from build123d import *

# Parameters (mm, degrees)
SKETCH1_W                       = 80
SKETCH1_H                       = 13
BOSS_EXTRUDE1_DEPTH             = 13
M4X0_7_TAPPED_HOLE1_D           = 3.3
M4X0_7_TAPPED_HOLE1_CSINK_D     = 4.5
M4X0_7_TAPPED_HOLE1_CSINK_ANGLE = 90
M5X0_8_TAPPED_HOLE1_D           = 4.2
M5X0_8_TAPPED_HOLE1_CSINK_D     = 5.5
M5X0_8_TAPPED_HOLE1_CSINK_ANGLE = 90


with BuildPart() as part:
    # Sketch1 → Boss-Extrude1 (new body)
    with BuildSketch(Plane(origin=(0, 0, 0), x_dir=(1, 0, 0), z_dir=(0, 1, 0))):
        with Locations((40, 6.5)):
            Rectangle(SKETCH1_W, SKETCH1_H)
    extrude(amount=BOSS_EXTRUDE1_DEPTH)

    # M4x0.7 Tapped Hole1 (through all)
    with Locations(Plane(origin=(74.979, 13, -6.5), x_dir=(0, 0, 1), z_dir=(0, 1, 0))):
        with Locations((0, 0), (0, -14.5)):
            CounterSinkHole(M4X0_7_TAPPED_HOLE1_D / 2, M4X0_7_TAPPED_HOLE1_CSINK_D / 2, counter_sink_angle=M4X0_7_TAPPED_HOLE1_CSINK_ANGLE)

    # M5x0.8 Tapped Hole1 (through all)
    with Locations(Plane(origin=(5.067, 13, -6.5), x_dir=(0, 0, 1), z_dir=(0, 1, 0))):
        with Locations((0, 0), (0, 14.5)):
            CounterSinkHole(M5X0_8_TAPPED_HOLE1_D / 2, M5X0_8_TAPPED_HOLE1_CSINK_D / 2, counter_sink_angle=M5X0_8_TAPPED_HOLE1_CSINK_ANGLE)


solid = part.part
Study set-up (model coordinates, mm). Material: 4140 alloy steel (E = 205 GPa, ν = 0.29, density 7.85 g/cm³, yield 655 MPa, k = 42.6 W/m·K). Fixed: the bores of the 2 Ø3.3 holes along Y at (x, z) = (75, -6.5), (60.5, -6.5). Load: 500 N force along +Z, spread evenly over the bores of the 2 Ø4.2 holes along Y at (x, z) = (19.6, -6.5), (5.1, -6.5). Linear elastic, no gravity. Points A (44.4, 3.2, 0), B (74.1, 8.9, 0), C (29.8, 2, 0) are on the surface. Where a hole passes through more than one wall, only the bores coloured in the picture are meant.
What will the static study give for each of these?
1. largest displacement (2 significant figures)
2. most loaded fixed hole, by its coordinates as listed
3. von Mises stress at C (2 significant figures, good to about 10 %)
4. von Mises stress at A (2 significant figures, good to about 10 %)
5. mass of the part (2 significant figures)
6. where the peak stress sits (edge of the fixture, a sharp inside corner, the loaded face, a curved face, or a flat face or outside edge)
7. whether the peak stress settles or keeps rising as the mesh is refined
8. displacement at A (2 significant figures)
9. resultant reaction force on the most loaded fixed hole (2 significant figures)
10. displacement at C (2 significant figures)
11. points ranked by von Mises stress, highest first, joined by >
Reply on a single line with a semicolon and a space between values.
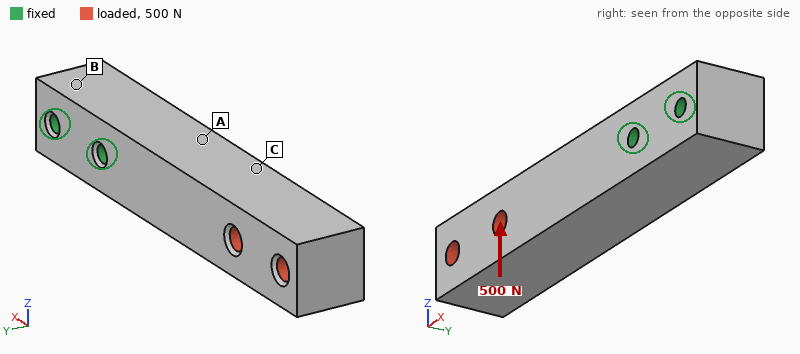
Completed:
70 µm; (60.5, -6.5); 24 MPa; 44 MPa; 100 g; edge of the fixture; keeps rising; 12 µm; 1.5 kN; 28 µm; A > C > B
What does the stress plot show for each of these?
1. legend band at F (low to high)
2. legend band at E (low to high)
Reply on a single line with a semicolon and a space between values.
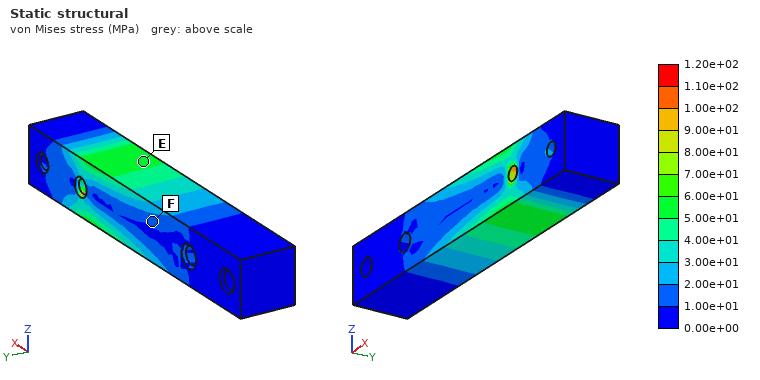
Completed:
1.00e+01 to 2.00e+01 MPa; 5.00e+01 to 6.00e+01 MPa
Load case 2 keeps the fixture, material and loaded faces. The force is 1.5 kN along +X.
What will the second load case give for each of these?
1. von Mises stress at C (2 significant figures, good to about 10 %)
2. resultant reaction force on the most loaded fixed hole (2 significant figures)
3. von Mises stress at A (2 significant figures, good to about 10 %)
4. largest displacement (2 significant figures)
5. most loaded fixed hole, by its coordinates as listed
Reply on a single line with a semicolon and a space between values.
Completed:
10 MPa; 1.3 kN; 9.6 MPa; 3.3 µm; (60.5, -6.5)
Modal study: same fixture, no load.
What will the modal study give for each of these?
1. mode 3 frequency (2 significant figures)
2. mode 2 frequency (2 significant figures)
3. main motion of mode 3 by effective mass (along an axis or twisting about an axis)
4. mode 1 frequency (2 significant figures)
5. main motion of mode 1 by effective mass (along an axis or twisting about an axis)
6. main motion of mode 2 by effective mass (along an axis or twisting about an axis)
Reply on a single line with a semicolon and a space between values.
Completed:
12 kHz; 2900 Hz; twisting about X; 2600 Hz; along Z; along Y
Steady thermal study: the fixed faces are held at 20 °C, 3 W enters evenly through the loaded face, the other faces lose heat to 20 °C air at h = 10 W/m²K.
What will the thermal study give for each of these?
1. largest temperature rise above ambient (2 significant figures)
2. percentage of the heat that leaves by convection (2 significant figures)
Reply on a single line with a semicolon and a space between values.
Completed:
19 K; 12 %
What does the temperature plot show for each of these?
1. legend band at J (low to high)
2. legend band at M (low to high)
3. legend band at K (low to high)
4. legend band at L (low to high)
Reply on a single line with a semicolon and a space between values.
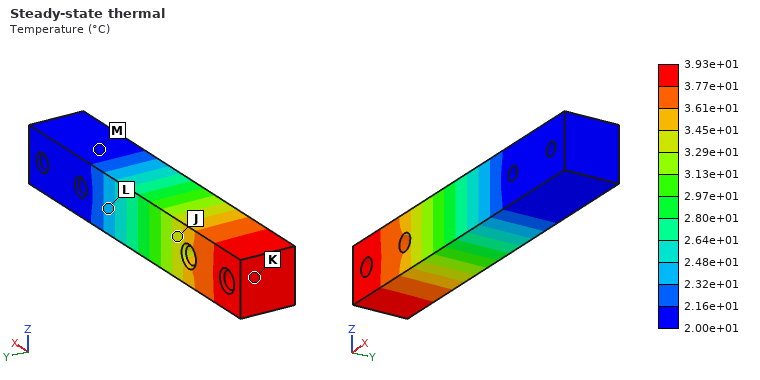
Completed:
3.29e+01 to 3.45e+01 °C; 2.00e+01 to 2.16e+01 °C; 3.77e+01 to 3.93e+01 °C; 2.32e+01 to 2.48e+01 °C
